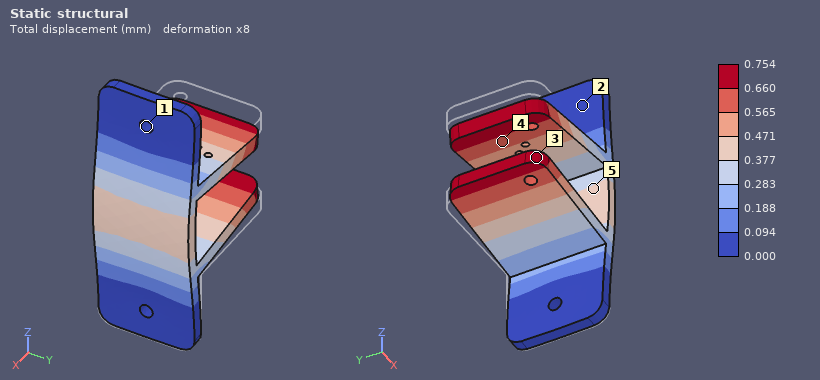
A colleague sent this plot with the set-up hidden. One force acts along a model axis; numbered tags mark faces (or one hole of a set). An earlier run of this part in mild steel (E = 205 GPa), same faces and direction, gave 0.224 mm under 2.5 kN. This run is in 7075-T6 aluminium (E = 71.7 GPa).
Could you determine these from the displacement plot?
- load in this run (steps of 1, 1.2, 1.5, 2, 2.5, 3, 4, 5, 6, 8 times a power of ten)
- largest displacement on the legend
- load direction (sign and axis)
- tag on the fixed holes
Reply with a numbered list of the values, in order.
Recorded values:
1. 3 kN
2. 0.754 mm
3. +X
4. 1
